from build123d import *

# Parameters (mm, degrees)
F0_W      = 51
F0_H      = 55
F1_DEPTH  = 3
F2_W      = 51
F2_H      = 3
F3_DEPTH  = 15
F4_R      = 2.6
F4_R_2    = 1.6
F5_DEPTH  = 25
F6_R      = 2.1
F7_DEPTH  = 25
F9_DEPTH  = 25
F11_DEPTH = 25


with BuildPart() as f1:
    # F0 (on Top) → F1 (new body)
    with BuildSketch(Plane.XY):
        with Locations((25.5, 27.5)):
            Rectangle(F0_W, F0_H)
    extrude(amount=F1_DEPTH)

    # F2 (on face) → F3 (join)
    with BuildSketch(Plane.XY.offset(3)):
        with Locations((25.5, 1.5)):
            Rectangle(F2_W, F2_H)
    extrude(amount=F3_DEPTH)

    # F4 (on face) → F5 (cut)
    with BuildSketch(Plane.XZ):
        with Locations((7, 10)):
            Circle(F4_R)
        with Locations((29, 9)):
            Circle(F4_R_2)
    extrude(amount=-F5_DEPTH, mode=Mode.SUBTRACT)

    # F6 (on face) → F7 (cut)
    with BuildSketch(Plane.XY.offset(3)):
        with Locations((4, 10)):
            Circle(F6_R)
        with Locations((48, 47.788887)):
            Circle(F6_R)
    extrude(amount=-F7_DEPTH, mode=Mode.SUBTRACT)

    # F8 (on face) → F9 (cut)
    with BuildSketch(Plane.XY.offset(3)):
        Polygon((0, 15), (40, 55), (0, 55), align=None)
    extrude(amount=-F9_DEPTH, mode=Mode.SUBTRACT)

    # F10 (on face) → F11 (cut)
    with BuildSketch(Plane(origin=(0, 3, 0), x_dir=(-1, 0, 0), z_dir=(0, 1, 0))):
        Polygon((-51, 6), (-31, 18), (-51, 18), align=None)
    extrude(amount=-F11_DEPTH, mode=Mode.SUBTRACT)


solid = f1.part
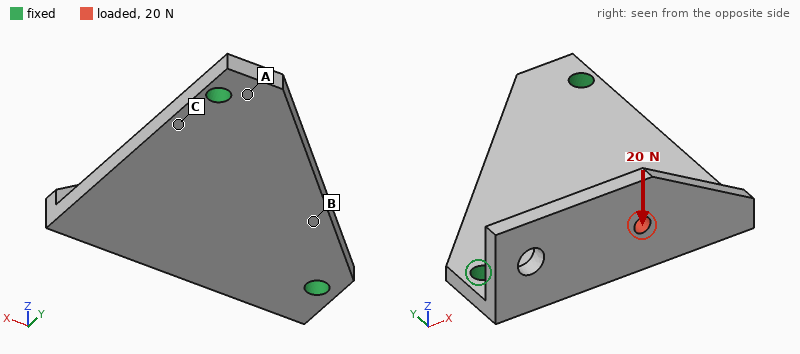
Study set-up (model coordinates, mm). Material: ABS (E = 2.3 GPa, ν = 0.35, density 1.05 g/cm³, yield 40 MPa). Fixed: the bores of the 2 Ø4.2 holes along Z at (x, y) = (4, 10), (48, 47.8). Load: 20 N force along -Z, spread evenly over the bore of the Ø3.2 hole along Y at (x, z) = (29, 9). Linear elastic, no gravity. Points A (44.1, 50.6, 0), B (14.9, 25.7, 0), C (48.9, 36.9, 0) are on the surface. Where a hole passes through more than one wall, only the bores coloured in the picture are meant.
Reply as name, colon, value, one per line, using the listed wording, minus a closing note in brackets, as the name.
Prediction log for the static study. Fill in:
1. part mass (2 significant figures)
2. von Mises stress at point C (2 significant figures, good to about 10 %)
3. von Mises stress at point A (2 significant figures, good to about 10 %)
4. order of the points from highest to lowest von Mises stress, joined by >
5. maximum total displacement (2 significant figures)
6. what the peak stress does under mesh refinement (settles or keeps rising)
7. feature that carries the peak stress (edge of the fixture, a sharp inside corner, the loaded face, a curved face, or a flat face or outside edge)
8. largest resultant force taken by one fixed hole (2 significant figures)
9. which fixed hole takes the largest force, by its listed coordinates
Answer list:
part mass: 8.2 g
von Mises stress at point C: 3.4 MPa
von Mises stress at point A: 2.1 MPa
order of the points from highest to lowest von Mises stress, joined by >: C > A > B
maximum total displacement: 0.86 mm
what the peak stress does under mesh refinement: keeps rising
feature that carries the peak stress: edge of the fixture
largest resultant force taken by one fixed hole: 17 N
which fixed hole takes the largest force, by its listed coordinates: (4, 10)
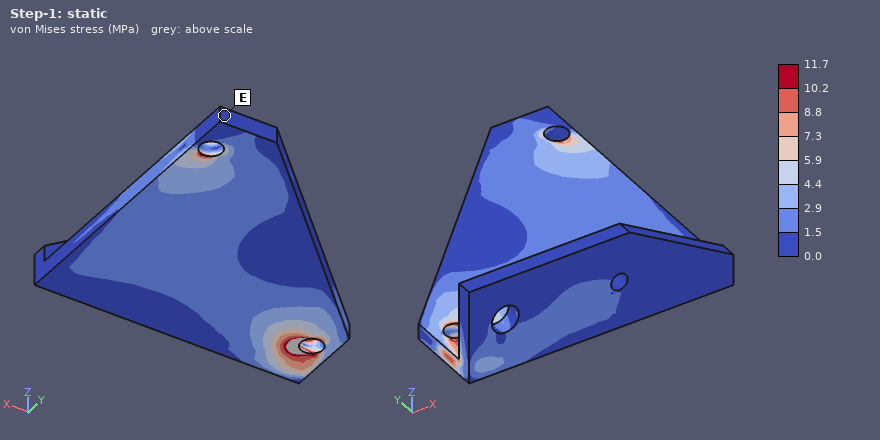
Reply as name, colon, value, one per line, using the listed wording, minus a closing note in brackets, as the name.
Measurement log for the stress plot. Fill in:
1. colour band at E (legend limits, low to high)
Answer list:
colour band at E: 0.0 to 1.5 MPa
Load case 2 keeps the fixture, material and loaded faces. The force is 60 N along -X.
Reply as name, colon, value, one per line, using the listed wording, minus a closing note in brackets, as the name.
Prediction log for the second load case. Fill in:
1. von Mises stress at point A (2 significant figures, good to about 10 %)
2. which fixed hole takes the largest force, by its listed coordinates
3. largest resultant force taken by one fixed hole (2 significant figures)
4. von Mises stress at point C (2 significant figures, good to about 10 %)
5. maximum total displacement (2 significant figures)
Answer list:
von Mises stress at point A: 1.9 MPa
which fixed hole takes the largest force, by its listed coordinates: (4, 10)
largest resultant force taken by one fixed hole: 57 N
von Mises stress at point C: 3.5 MPa
maximum total displacement: 0.77 mm
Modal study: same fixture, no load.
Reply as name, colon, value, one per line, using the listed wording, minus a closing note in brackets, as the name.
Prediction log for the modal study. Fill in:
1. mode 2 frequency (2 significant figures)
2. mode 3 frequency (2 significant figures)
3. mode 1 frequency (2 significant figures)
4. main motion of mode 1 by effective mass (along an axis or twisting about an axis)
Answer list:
mode 2 frequency: 1300 Hz
mode 3 frequency: 1800 Hz
mode 1 frequency: 510 Hz
main motion of mode 1 by effective mass: along Z
